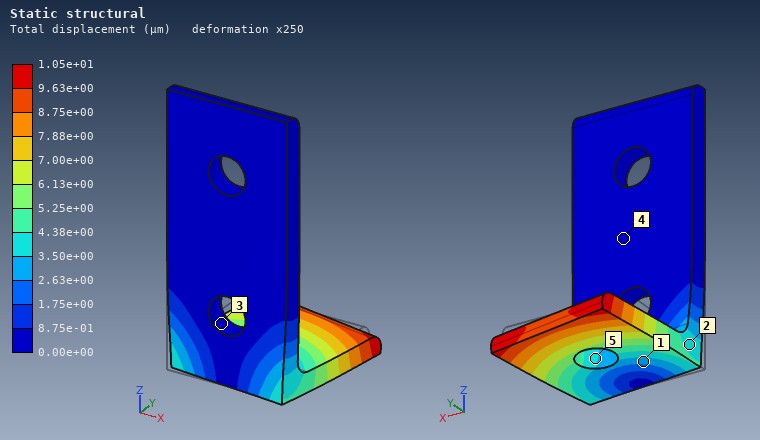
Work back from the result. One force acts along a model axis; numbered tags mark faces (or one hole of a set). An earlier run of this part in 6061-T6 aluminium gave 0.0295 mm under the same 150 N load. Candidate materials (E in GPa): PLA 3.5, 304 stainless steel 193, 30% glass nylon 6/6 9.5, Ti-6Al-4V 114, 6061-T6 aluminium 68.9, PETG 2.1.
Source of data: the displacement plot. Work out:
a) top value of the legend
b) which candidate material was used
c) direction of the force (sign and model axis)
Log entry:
1.05e+01 µm
304 stainless steel
+X
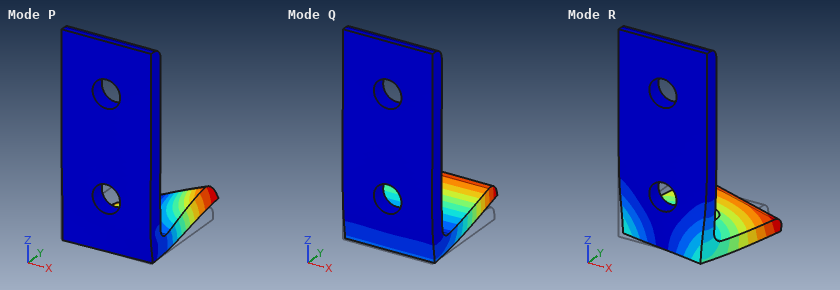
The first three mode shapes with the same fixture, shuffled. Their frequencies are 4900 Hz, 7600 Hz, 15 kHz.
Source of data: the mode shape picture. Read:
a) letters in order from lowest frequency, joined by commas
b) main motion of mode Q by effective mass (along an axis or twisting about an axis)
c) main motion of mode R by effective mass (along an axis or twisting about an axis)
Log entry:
Q, R, P
along Z
along X
